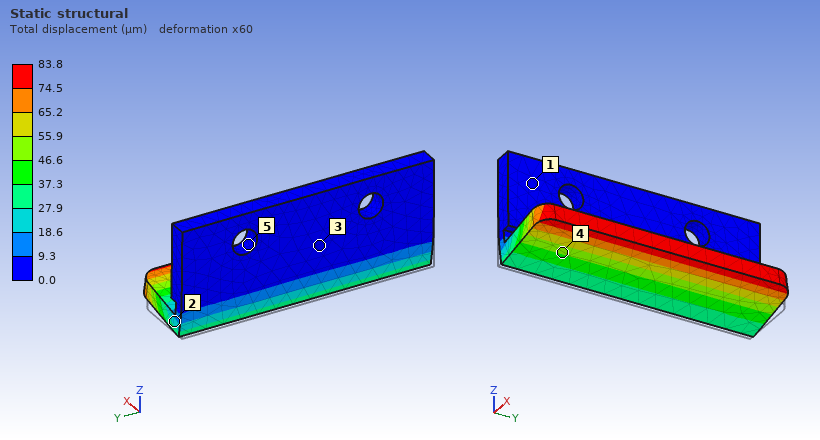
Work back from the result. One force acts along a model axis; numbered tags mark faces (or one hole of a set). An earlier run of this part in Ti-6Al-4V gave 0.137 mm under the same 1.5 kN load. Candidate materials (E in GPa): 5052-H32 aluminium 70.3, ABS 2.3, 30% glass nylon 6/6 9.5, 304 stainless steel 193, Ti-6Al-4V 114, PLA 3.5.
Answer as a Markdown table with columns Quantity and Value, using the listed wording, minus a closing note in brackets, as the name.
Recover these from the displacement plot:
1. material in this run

| Quantity | Value |
|---|---|
| material in this run | 304 stainless steel |
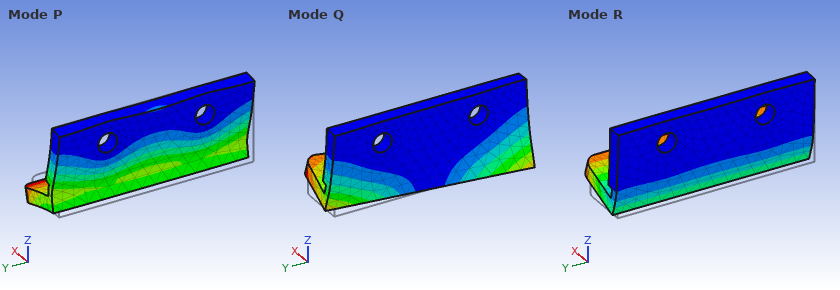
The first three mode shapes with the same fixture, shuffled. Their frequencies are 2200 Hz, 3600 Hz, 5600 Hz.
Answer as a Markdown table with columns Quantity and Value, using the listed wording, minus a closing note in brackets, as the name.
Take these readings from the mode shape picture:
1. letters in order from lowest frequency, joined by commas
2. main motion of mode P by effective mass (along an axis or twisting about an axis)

| Quantity | Value |
|---|---|
| letters in order from lowest frequency, joined by commas | R, Q, P |
| main motion of mode P by effective mass | along X |
